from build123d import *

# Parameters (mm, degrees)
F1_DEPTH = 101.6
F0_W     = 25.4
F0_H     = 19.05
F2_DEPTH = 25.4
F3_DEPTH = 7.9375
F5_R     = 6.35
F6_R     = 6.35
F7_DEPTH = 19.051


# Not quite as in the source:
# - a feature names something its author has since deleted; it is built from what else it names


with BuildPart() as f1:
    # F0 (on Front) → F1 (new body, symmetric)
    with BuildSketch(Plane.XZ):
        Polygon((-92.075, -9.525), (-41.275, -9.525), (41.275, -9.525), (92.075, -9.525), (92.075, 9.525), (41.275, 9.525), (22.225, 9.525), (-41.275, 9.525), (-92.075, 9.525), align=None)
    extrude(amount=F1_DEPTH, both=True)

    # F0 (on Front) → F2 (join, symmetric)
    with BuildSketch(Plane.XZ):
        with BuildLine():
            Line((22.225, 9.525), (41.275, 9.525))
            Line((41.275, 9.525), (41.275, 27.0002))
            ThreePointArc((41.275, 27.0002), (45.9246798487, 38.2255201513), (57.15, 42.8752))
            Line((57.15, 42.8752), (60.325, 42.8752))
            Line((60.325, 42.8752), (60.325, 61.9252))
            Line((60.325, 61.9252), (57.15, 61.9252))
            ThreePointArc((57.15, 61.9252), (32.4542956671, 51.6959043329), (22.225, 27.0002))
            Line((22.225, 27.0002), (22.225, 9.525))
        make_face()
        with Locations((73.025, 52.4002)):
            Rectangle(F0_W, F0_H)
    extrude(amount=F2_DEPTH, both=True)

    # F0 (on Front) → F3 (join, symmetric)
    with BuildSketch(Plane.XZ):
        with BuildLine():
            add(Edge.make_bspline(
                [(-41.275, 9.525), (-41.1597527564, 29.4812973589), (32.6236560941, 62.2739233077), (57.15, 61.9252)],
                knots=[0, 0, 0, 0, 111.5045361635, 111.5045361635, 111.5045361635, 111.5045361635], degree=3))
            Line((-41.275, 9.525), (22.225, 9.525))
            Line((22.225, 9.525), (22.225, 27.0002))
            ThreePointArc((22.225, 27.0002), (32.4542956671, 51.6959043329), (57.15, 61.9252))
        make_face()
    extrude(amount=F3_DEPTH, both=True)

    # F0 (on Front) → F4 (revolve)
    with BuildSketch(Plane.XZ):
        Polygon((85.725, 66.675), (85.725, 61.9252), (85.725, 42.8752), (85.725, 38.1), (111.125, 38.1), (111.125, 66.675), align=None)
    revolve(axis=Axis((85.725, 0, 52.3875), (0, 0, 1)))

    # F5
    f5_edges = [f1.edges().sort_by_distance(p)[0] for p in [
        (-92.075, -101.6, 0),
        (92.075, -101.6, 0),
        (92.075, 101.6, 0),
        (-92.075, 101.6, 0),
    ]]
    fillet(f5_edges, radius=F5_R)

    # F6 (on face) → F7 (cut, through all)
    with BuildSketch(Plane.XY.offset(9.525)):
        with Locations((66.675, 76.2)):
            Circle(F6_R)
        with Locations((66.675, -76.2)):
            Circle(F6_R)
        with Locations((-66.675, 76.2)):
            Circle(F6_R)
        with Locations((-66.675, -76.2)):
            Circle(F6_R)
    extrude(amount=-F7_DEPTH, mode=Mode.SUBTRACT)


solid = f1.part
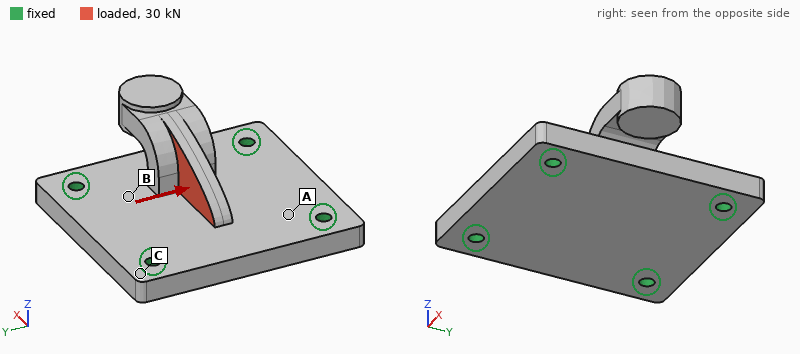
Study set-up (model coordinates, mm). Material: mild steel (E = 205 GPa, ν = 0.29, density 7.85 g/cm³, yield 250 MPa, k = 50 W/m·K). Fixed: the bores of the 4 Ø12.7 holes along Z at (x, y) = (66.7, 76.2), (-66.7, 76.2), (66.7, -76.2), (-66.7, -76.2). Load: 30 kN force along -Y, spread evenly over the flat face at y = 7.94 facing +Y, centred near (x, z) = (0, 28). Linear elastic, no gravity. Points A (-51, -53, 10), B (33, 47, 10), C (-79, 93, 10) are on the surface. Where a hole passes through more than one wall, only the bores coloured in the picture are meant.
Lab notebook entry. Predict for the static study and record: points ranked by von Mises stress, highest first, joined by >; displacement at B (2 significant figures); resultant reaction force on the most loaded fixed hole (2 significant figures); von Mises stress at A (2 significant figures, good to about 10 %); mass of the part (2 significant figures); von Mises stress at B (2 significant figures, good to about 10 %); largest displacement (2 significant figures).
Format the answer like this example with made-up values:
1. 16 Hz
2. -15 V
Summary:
1. B > A > C
2. 8.6 µm
3. 9.5 kN
4. 11 MPa
5. 6.7 kg
6. 20 MPa
7. 47 µm
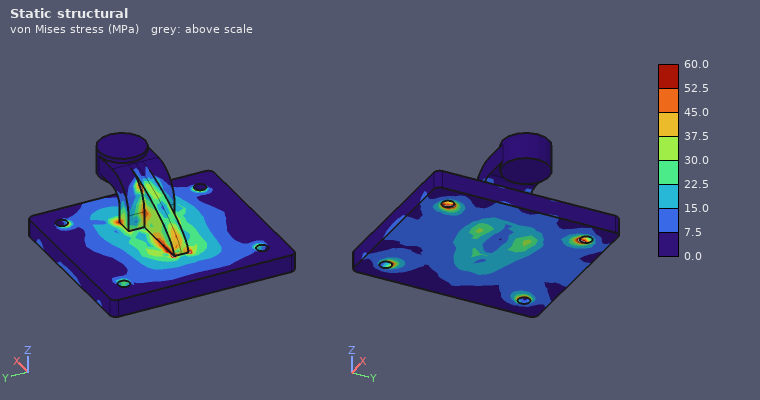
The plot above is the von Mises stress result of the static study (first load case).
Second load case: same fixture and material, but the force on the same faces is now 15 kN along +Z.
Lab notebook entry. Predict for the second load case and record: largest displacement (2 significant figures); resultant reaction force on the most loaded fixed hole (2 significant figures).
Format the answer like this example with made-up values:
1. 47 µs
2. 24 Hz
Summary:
1. 29 µm
2. 4.4 kN
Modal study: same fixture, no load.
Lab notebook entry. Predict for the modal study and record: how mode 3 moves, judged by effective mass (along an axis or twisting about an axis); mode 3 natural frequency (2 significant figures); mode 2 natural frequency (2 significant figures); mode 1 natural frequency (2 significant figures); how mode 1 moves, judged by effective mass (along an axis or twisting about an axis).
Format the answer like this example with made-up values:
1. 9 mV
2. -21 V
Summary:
1. along Z
2. 2800 Hz
3. 1900 Hz
4. 1600 Hz
5. along Z
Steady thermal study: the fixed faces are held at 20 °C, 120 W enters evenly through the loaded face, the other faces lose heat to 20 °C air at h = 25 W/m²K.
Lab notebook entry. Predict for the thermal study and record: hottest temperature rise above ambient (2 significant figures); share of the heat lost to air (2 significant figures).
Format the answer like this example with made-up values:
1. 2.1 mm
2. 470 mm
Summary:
1. 68 K
2. 33 %
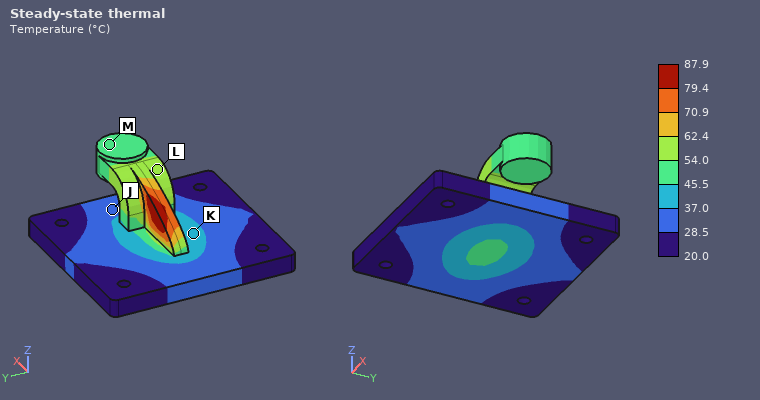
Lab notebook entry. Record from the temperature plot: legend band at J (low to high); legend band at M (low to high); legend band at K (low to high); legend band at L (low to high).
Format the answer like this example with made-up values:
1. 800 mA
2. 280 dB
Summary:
1. 28.5 to 37.0 °C
2. 45.5 to 54.0 °C
3. 37.0 to 45.5 °C
4. 54.0 to 62.4 °C
